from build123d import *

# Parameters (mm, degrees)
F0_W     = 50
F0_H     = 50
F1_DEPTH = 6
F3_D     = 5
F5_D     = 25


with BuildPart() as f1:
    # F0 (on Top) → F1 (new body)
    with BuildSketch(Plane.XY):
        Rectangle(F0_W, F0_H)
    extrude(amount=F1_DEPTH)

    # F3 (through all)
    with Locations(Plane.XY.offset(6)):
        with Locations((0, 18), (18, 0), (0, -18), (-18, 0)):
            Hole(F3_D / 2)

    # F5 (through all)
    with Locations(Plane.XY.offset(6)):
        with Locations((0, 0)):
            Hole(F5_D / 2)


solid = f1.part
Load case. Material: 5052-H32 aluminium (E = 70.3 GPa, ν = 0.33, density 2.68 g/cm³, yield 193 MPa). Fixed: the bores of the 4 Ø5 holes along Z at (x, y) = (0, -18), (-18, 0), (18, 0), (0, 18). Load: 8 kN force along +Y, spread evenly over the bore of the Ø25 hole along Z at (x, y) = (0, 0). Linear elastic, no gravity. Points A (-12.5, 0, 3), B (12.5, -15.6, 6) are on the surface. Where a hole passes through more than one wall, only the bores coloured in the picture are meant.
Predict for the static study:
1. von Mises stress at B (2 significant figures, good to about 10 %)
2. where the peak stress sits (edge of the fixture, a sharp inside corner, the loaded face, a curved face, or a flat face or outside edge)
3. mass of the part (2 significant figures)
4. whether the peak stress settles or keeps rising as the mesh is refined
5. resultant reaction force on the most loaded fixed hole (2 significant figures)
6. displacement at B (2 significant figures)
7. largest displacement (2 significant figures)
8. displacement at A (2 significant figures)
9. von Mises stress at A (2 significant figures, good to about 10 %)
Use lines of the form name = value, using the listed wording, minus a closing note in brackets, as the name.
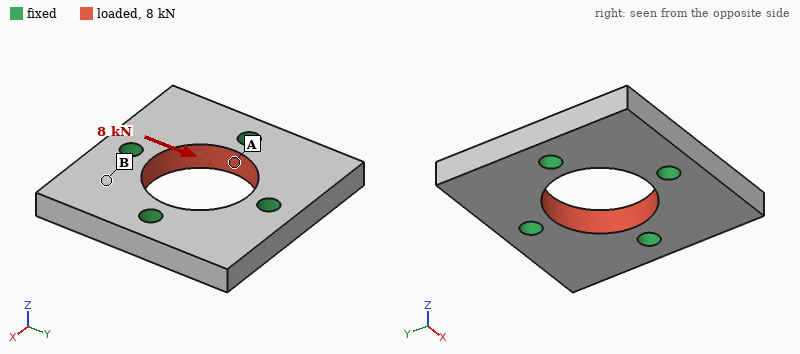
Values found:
von Mises stress at B = 9.1 MPa
where the peak stress sits = edge of the fixture
mass of the part = 31 g
whether the peak stress settles or keeps rising as the mesh is refined = keeps rising
resultant reaction force on the most loaded fixed hole = 2.1 kN
displacement at B = 2.7 µm
largest displacement = 4.1 µm
displacement at A = 3.1 µm
von Mises stress at A = 29 MPa
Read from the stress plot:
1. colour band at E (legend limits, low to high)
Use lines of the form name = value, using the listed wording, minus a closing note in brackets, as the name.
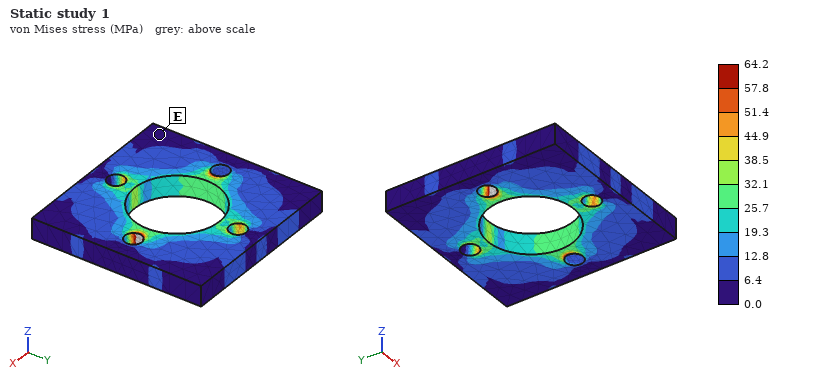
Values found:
colour band at E = 0.0 to 6.4 MPa
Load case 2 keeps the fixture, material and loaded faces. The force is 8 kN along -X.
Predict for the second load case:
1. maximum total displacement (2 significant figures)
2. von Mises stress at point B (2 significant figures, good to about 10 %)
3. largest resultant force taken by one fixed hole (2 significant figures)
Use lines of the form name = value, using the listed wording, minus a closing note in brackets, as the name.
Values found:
maximum total displacement = 4.1 µm
von Mises stress at point B = 9.2 MPa
largest resultant force taken by one fixed hole = 2.1 kN
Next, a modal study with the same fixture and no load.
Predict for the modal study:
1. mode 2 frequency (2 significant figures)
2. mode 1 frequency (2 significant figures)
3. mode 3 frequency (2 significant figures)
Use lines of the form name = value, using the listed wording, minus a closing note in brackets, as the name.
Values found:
mode 2 frequency = 14 kHz
mode 1 frequency = 14 kHz
mode 3 frequency = 14 kHz
